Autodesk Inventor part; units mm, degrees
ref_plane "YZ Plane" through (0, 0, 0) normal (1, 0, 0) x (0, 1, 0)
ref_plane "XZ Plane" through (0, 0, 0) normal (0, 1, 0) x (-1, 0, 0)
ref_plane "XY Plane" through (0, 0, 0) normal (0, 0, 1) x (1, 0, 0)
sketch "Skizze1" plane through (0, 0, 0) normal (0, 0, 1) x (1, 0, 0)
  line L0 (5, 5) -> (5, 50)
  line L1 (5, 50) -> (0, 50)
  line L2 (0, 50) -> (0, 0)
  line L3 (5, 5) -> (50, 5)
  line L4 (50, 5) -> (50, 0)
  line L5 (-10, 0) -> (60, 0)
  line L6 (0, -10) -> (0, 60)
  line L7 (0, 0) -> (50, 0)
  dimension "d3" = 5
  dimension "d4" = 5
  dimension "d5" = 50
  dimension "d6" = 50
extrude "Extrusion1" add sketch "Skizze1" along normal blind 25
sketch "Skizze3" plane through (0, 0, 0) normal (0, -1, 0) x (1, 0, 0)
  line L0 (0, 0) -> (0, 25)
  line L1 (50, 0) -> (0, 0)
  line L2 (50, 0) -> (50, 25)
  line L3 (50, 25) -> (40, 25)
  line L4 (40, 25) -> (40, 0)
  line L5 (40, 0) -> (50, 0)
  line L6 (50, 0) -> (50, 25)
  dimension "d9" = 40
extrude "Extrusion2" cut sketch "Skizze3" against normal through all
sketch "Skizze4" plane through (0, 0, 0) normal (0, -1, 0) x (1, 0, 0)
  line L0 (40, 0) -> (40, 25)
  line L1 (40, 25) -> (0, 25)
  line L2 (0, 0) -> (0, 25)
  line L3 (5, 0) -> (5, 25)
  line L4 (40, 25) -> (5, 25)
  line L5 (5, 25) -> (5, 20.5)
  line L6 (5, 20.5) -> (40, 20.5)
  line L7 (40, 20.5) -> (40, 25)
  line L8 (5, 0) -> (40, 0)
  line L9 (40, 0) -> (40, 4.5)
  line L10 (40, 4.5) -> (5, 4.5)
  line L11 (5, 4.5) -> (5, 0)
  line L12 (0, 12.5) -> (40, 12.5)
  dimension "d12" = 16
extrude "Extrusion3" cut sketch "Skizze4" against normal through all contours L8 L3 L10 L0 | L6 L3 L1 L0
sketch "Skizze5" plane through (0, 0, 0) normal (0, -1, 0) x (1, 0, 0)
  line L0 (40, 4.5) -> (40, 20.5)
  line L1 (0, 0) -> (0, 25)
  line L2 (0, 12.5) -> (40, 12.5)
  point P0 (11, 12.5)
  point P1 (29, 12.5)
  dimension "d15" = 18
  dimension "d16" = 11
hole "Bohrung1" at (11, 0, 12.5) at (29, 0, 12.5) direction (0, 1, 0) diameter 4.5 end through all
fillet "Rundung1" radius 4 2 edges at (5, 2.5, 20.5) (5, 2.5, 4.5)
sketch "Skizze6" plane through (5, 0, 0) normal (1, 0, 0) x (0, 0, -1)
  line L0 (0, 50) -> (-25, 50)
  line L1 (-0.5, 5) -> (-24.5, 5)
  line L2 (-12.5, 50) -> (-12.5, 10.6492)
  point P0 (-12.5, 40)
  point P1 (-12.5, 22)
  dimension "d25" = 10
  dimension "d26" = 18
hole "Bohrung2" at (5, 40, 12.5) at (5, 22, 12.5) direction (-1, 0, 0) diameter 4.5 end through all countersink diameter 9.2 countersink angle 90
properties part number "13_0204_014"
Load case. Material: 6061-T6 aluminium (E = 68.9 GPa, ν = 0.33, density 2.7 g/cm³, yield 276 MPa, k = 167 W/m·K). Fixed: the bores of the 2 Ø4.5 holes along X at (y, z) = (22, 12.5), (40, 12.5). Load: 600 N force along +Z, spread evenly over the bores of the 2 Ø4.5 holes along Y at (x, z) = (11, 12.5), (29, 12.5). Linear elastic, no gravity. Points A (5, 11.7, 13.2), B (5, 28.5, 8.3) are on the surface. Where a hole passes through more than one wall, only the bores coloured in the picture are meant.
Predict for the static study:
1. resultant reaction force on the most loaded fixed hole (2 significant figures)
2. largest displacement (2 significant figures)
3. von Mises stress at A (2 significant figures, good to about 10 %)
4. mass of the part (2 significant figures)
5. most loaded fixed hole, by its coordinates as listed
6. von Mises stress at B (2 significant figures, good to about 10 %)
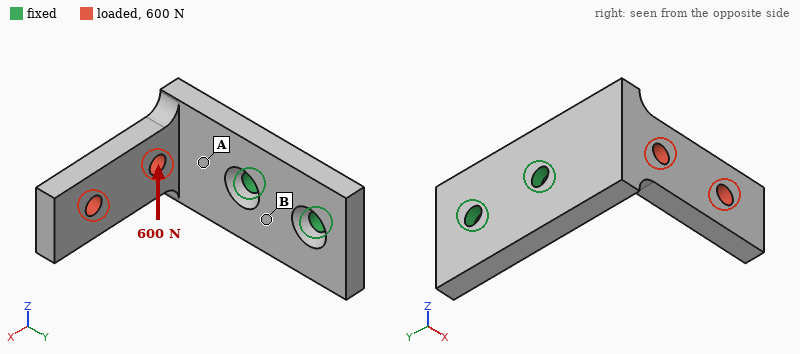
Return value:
1.0 kN
0.43 mm
100 MPa
23 g
(22, 12.5)
38 MPa
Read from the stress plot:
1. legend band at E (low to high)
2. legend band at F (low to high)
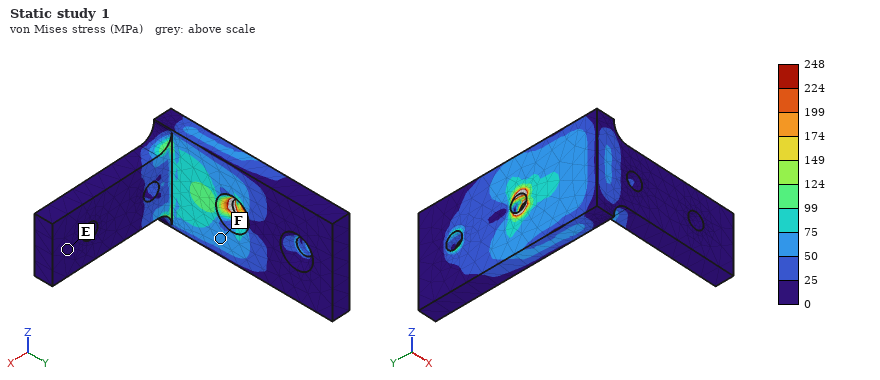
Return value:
0 to 25 MPa
50 to 75 MPa
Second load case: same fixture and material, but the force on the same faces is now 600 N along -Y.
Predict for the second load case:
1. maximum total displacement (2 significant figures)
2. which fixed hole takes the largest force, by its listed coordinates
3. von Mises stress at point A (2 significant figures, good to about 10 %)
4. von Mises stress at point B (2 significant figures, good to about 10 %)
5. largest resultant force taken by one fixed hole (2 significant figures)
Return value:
0.80 mm
(40, 12.5)
93 MPa
35 MPa
760 N
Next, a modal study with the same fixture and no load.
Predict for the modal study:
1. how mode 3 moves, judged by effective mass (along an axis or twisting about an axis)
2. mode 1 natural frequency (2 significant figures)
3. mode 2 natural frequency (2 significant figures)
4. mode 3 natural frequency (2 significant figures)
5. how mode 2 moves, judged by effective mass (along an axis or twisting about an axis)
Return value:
along X
1700 Hz
2400 Hz
4900 Hz
along Z
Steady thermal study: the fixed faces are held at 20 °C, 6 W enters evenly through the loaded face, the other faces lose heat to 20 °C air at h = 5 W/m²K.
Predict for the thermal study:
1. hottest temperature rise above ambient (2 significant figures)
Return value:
15 K
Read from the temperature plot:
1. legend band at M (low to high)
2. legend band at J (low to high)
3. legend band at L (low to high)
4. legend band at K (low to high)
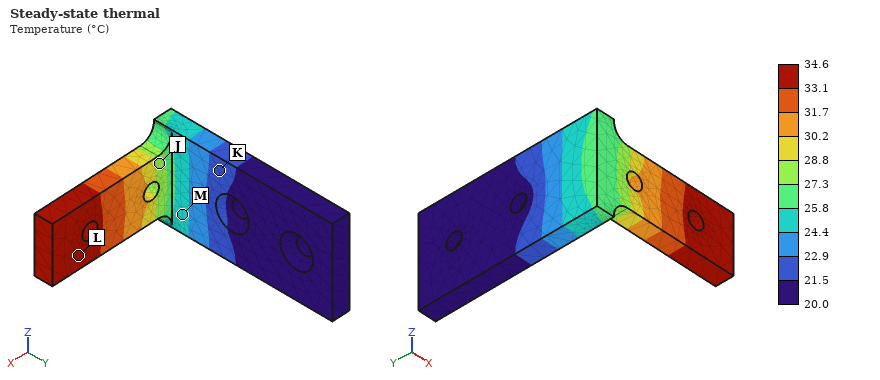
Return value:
24.4 to 25.8 °C
27.3 to 28.8 °C
33.1 to 34.6 °C
21.5 to 22.9 °C
